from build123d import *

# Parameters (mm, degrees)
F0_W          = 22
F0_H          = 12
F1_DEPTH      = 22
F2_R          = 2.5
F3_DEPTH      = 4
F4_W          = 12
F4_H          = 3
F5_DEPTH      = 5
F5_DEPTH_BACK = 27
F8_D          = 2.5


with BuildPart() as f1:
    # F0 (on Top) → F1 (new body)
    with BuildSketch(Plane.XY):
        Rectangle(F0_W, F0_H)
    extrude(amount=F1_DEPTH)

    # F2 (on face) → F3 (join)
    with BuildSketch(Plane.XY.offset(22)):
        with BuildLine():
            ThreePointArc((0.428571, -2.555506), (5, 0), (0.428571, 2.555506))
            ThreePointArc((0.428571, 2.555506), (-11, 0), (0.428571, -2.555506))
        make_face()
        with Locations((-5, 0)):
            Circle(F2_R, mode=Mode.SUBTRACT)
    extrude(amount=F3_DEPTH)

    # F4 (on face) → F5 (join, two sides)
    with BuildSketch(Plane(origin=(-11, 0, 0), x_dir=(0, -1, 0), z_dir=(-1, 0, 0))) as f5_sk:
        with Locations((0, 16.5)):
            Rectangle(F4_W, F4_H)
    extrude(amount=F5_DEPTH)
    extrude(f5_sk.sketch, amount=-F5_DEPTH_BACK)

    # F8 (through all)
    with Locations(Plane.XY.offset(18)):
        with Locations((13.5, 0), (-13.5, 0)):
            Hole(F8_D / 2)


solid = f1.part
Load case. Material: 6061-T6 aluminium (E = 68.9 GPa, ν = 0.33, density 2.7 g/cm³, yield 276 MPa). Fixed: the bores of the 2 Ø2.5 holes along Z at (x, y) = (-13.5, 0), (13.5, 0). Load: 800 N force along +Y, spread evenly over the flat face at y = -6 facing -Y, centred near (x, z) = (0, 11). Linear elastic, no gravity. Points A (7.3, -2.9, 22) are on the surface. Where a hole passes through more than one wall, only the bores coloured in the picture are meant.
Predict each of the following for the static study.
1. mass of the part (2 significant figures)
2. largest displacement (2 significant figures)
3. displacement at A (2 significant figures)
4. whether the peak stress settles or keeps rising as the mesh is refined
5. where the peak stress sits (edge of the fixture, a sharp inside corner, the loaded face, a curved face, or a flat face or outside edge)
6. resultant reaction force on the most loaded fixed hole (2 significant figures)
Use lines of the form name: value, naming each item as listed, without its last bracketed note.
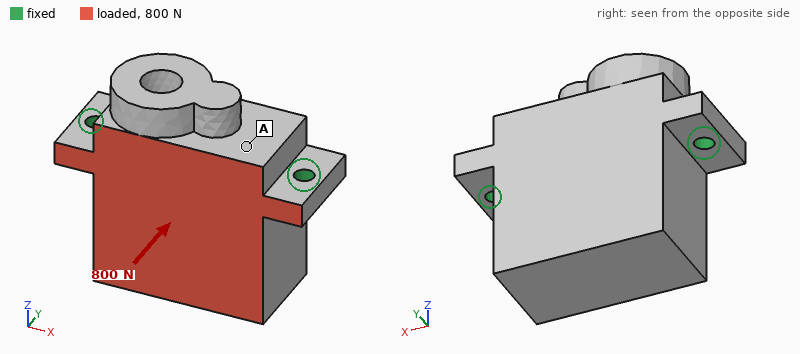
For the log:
mass of the part: 18 g
largest displacement: 47 µm
displacement at A: 12 µm
whether the peak stress settles or keeps rising as the mesh is refined: keeps rising
where the peak stress sits: edge of the fixture
resultant reaction force on the most loaded fixed hole: 400 N
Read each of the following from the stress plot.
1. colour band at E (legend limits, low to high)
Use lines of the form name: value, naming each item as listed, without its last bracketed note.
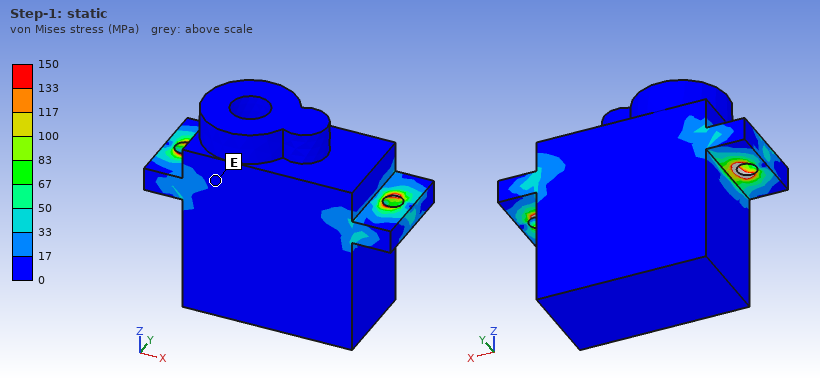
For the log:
colour band at E: 0 to 17 MPa
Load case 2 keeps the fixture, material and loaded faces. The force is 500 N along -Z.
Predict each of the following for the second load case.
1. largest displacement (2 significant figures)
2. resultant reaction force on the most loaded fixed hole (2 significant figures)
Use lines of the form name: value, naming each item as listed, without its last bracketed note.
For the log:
largest displacement: 31 µm
resultant reaction force on the most loaded fixed hole: 250 N
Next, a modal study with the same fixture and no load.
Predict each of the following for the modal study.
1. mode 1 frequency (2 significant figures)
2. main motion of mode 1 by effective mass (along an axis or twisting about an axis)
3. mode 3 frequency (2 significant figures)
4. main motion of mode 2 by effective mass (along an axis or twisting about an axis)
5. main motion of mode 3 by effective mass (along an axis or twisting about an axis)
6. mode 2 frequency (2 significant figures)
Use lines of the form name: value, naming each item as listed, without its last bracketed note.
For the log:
mode 1 frequency: 5500 Hz
main motion of mode 1 by effective mass: along Y
mode 3 frequency: 20 kHz
main motion of mode 2 by effective mass: along Z
main motion of mode 3 by effective mass: along X
mode 2 frequency: 19 kHz
